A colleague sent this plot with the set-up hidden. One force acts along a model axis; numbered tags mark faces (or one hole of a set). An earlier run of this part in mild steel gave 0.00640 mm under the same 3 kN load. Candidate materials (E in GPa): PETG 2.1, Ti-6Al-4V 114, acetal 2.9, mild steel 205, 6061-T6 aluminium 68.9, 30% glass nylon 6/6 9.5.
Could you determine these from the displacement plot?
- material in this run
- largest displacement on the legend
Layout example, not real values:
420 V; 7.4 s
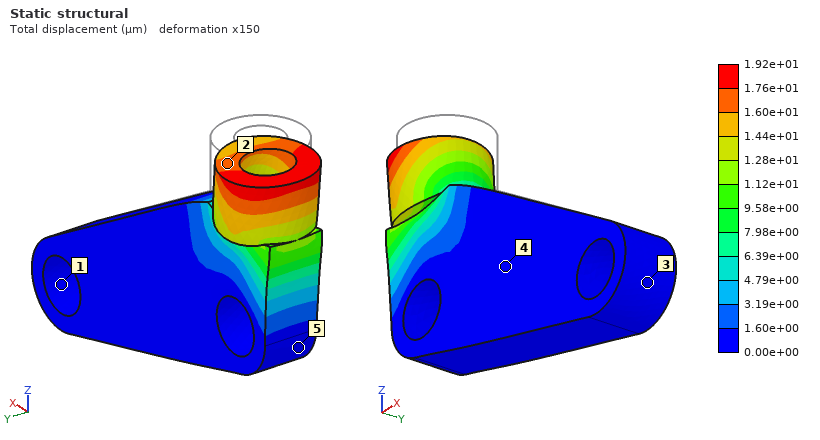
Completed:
6061-T6 aluminium; 1.92e+01 µm
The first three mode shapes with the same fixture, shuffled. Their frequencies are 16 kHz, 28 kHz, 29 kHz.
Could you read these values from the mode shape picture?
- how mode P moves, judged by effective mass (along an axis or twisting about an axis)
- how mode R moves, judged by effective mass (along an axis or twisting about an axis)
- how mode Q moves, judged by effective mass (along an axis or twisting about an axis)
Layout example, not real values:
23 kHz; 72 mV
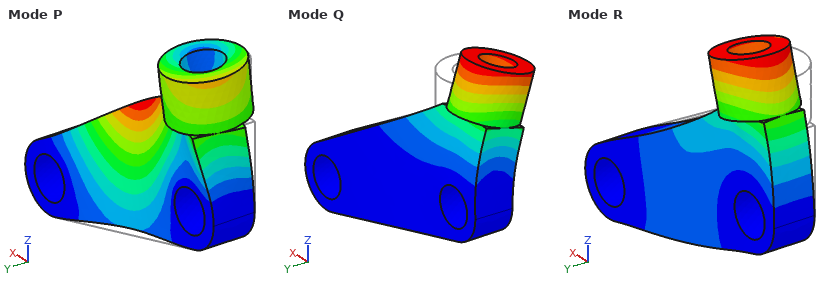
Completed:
along Y; along X; along Y
